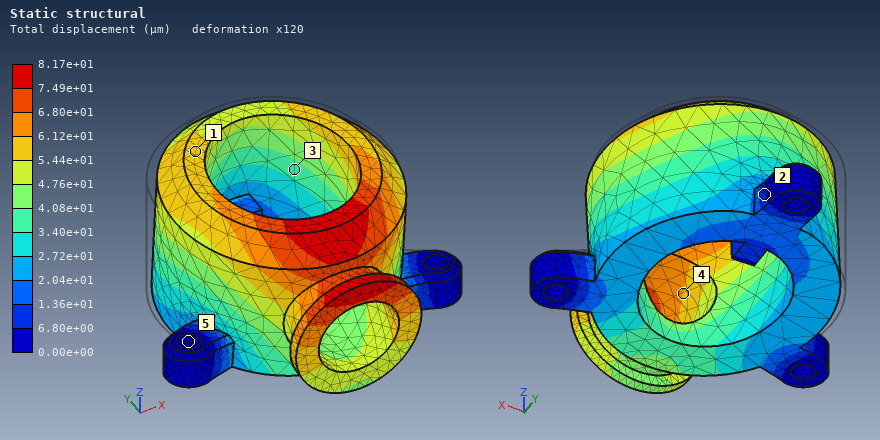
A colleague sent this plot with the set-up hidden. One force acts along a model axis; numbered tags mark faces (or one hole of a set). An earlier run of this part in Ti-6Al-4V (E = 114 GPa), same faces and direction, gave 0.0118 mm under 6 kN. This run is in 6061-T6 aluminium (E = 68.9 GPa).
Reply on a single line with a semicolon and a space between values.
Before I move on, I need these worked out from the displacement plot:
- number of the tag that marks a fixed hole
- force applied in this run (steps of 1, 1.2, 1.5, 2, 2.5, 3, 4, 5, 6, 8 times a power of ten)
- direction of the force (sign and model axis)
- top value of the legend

5; 25 kN; -Y; 8.17e+01 µm
